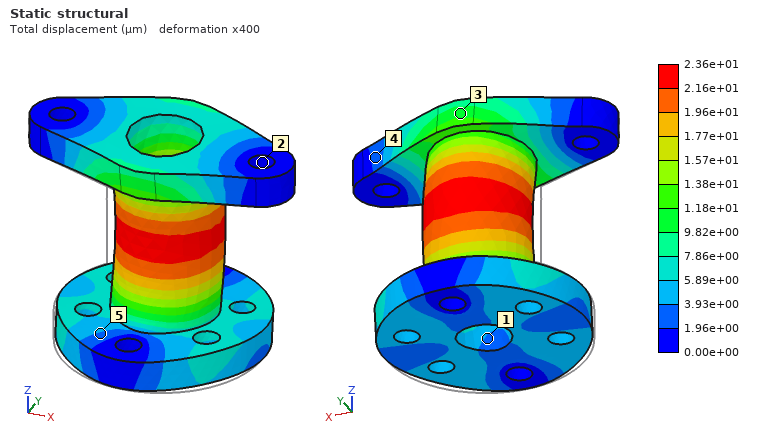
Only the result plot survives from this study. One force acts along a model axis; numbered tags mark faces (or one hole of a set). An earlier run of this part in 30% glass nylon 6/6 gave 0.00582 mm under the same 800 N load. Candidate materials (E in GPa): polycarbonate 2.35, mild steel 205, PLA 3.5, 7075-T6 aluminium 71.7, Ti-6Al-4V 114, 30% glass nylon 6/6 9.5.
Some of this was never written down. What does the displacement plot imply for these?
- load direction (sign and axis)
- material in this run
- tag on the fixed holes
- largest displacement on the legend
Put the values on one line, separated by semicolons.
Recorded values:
+Y; polycarbonate; 2; 2.36e+01 µm
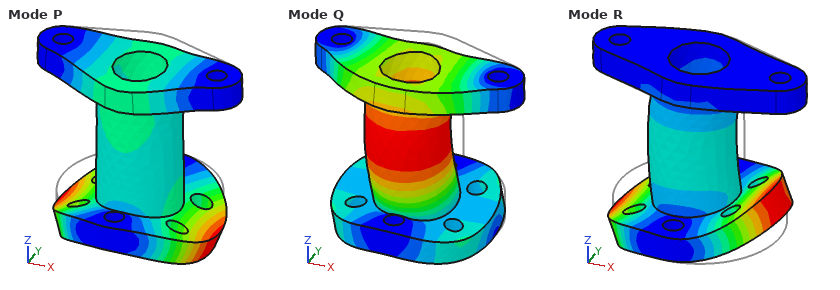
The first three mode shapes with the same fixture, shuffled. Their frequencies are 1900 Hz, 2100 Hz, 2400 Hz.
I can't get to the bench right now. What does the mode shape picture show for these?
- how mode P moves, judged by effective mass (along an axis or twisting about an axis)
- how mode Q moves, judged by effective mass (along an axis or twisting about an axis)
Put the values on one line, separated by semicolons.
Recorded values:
along Z; along Y
